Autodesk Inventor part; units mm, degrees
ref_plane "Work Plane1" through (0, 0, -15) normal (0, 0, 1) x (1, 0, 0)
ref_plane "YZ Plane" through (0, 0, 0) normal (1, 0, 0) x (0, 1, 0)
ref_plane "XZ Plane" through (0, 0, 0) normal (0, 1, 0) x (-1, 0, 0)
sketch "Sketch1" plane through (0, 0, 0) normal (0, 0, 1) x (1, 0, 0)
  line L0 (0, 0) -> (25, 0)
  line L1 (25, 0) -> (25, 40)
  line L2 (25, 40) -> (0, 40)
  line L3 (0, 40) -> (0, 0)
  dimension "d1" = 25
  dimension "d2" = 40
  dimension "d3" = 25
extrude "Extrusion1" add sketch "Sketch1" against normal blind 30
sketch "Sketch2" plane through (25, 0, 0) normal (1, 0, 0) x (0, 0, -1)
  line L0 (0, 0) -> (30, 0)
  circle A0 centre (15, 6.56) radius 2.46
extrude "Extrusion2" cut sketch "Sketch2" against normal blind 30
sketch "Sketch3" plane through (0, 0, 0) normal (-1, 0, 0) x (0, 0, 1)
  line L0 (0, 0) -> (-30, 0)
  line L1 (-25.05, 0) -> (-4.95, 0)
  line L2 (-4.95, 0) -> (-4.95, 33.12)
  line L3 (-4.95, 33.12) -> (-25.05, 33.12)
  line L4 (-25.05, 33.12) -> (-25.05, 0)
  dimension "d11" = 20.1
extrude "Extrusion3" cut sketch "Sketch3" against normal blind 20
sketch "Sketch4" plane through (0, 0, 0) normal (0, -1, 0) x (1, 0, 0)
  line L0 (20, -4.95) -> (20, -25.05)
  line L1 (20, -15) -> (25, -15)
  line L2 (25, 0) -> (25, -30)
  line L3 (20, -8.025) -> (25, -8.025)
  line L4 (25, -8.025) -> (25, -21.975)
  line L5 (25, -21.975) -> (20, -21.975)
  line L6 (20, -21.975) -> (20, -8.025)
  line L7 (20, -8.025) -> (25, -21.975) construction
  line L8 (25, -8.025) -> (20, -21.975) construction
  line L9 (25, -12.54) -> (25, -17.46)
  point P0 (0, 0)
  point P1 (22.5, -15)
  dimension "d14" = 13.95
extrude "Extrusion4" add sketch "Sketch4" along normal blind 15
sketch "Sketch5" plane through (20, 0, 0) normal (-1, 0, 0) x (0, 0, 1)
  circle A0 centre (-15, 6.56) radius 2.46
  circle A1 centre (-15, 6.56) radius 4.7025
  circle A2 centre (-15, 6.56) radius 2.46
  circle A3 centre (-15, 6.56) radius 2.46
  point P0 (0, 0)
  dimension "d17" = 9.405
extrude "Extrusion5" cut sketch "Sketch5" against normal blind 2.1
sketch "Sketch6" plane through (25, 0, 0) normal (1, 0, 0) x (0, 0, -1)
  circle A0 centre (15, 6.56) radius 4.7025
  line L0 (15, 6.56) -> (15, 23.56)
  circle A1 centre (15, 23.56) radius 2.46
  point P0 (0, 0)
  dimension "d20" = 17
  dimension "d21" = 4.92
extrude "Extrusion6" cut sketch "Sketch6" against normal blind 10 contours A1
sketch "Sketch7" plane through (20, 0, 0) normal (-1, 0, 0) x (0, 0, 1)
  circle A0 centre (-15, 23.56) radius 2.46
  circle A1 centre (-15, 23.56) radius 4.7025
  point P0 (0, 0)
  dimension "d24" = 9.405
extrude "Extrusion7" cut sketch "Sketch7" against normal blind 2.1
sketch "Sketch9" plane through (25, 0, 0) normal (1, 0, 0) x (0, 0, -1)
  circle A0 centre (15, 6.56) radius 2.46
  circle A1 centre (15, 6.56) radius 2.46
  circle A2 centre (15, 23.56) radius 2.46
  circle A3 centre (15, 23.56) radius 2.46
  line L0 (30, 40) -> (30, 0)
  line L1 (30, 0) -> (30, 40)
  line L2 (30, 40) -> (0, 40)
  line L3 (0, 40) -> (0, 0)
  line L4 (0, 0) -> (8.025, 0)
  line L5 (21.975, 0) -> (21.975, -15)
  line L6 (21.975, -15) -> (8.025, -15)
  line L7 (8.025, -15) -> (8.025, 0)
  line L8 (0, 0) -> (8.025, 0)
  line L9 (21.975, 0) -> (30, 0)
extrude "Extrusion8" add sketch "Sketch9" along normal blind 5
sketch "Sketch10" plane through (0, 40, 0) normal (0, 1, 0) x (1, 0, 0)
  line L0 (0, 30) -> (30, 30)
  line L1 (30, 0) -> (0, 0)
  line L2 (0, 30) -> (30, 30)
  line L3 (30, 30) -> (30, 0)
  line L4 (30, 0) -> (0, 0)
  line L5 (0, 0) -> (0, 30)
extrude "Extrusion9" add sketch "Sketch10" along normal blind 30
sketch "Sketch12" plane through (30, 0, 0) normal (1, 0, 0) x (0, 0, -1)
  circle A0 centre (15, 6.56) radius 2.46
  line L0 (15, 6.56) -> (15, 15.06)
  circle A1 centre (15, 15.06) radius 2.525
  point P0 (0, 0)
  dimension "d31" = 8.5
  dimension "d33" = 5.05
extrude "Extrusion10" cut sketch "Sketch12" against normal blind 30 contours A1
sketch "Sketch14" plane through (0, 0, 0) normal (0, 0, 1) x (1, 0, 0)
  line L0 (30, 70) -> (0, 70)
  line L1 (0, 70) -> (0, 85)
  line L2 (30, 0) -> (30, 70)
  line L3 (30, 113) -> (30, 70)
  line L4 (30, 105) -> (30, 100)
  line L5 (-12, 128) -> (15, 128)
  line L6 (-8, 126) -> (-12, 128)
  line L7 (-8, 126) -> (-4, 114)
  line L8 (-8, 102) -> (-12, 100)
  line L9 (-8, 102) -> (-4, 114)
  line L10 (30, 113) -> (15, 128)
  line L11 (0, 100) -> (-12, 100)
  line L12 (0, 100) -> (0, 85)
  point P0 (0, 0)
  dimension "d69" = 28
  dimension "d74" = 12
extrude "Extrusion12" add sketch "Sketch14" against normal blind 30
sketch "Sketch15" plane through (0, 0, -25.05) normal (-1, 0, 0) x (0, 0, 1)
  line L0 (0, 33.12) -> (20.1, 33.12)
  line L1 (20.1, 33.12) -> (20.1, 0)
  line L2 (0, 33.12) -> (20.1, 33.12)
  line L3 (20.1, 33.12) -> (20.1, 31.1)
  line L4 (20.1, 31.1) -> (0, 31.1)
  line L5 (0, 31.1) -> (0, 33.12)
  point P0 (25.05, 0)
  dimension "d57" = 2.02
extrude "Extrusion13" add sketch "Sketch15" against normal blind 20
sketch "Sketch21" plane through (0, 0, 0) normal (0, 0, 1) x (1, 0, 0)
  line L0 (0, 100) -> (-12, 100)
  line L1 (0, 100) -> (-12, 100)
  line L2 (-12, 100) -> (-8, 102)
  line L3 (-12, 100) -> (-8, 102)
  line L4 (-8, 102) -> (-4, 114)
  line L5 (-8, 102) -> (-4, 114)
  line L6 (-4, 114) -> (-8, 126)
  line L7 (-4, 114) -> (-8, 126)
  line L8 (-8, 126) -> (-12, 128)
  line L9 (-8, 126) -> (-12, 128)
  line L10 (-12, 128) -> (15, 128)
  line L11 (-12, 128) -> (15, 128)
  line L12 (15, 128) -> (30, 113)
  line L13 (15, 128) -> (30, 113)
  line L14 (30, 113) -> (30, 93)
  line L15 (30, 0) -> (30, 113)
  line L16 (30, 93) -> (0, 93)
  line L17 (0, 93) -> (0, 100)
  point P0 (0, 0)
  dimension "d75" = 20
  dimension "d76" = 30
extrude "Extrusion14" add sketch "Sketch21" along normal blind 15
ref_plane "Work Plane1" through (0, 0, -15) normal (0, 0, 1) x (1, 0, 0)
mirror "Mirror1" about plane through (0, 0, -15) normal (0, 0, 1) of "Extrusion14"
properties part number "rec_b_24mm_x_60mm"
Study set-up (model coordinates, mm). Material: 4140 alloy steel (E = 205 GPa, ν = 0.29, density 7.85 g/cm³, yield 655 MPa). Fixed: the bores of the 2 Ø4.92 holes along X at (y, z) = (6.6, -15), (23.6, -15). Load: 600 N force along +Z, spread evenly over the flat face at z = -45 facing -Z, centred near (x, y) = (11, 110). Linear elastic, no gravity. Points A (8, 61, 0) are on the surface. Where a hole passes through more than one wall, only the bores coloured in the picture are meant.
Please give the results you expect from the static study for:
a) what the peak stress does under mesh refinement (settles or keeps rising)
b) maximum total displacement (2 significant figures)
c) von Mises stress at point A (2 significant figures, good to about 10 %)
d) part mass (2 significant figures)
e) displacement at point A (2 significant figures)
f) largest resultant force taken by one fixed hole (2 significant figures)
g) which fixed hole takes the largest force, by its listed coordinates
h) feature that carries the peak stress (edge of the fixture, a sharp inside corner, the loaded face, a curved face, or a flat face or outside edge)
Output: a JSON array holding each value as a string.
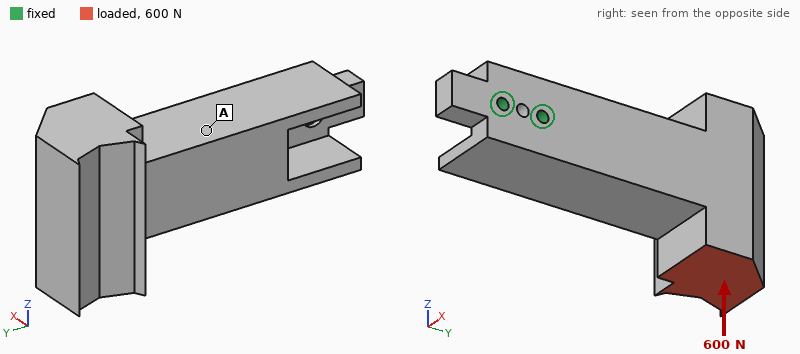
["keeps rising", "41 µm", "6.4 MPa", "1.1 kg", "13 µm", "2.8 kN", "(23.6, -15)", "edge of the fixture"]
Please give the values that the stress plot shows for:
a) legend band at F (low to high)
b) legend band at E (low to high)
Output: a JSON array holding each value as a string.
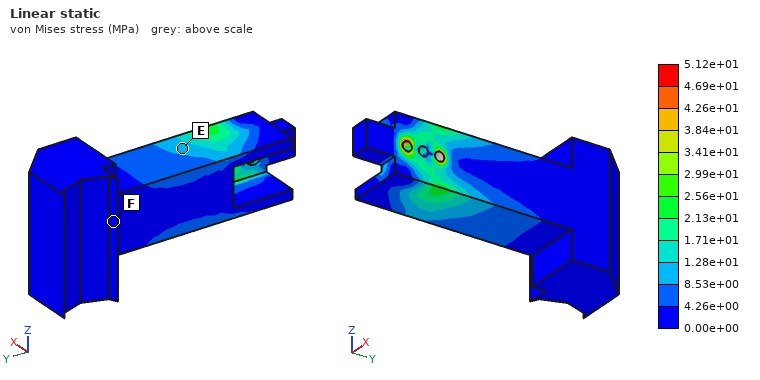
["0.00e+00 to 4.26e+00 MPa", "8.53e+00 to 1.28e+01 MPa"]
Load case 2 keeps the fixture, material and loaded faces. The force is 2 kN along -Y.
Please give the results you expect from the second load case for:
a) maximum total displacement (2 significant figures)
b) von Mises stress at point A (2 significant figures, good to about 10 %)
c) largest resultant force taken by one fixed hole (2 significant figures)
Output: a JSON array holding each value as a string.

["63 µm", "9.6 MPa", "3.1 kN"]
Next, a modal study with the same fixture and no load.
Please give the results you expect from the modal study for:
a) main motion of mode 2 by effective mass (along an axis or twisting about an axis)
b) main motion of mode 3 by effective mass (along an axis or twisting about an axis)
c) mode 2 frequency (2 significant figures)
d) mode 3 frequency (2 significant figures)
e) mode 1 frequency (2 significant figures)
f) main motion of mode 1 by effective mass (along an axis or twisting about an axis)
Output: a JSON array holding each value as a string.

["along Z", "twisting about Y", "870 Hz", "2000 Hz", "750 Hz", "along X"]
